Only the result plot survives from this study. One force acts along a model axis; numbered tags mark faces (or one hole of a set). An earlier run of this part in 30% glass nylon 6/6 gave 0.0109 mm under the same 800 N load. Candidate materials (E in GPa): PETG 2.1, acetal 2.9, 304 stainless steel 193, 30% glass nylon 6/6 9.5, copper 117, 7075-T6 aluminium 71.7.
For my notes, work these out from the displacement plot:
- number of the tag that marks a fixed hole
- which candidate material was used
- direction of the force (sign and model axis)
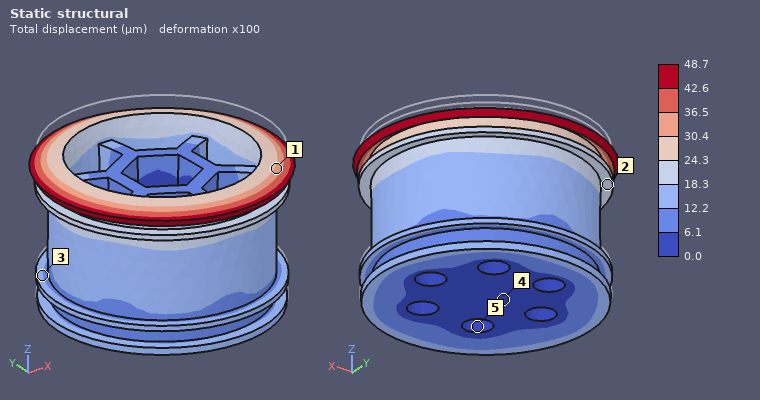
5
PETG
-Z
